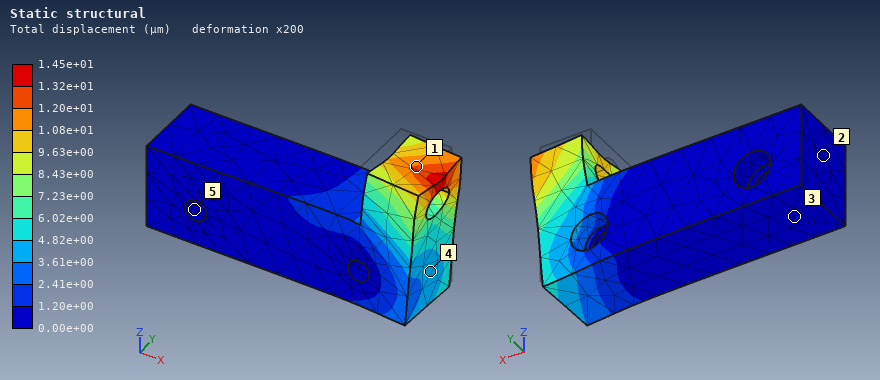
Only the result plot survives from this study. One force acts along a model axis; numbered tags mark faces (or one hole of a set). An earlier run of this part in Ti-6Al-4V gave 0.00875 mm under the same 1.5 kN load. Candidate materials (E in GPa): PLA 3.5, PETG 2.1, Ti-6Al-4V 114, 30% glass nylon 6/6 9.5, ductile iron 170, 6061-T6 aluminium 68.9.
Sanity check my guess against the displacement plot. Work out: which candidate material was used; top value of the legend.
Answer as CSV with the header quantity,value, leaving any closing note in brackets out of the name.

quantity,value
which candidate material was used,6061-T6 aluminium
top value of the legend,1.45e+01 µm
